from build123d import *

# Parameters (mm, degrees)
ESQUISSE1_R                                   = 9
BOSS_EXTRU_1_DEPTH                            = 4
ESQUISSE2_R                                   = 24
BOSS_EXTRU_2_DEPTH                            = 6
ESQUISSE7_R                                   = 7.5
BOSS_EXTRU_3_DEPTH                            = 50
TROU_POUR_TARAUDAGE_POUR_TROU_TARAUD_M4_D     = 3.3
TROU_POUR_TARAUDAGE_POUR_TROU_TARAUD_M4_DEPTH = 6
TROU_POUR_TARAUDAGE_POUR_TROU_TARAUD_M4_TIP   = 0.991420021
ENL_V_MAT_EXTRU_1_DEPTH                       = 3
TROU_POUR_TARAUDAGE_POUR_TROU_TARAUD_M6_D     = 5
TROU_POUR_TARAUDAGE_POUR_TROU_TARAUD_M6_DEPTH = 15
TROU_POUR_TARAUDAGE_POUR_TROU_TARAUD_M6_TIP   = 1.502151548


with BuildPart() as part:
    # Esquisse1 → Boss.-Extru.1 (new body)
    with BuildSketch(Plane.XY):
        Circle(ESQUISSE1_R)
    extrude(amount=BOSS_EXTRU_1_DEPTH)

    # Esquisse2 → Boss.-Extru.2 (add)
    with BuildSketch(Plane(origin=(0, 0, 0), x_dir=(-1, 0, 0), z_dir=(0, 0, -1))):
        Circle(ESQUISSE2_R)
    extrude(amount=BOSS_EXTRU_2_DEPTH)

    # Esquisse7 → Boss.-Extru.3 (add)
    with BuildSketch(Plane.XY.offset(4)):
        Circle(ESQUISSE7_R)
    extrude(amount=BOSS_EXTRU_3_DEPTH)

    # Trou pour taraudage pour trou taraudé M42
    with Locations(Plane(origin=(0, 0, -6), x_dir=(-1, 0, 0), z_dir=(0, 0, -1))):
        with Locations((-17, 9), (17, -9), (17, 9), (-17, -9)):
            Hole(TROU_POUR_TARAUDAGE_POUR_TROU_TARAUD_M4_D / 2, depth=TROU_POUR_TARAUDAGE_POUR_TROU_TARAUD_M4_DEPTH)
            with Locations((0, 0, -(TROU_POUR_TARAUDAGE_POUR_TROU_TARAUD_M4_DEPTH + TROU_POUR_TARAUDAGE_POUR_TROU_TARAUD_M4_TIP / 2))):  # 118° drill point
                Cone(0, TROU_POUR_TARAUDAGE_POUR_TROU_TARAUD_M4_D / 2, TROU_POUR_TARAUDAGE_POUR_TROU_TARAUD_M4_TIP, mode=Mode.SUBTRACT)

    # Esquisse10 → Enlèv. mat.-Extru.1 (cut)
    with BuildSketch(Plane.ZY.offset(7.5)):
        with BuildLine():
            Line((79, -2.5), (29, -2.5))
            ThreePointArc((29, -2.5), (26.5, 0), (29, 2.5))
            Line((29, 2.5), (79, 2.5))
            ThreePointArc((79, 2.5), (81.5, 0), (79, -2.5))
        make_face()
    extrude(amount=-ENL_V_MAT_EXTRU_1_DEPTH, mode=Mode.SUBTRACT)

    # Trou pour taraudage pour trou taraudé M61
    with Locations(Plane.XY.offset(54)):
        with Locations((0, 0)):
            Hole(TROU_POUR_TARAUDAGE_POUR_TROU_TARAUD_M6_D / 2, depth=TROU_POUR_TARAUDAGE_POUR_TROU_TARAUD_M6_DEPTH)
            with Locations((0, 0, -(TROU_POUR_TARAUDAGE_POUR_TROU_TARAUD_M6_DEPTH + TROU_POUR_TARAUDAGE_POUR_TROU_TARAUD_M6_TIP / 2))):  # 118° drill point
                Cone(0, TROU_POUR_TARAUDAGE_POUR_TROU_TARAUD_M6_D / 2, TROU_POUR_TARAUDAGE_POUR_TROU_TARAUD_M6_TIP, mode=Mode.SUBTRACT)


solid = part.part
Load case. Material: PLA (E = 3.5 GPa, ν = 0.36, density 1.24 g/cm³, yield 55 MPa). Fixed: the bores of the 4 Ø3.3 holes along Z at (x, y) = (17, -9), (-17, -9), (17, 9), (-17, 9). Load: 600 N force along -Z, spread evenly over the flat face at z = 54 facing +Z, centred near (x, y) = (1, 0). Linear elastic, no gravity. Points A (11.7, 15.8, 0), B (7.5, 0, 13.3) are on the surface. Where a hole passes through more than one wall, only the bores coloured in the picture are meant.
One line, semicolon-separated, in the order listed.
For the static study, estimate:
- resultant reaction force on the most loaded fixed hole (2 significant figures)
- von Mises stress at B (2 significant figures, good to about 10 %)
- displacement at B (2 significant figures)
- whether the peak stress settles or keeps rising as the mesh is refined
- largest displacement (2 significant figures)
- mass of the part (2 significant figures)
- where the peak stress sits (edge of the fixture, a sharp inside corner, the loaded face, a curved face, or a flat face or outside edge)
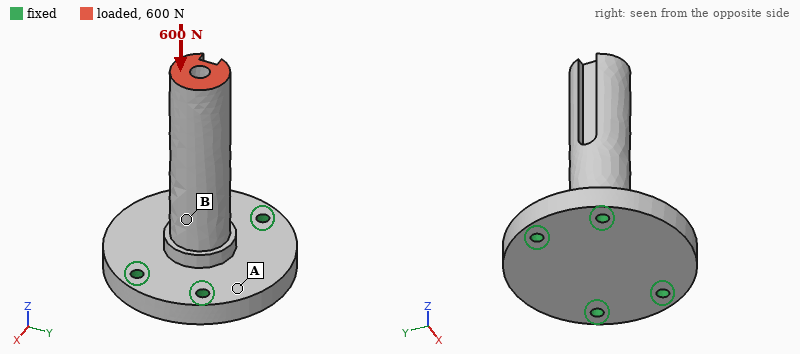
160 N; 4.5 MPa; 0.065 mm; keeps rising; 0.13 mm; 25 g; edge of the fixture
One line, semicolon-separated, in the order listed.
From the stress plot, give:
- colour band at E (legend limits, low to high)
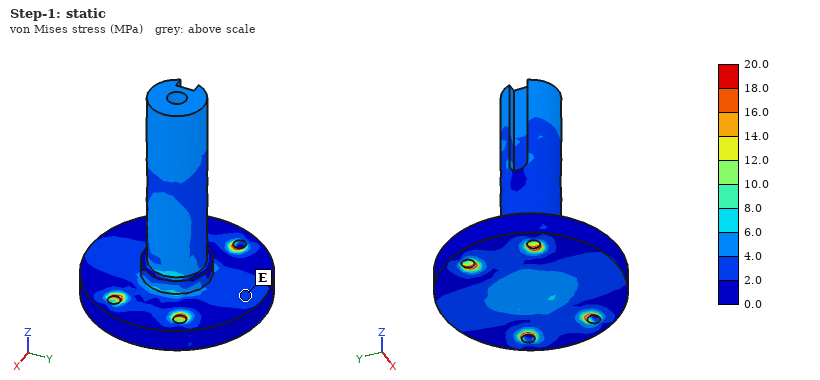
2.0 to 4.0 MPa
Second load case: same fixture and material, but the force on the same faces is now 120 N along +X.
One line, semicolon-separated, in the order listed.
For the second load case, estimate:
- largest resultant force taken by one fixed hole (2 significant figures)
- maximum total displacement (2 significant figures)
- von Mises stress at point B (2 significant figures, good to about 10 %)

130 N; 0.95 mm; 15 MPa
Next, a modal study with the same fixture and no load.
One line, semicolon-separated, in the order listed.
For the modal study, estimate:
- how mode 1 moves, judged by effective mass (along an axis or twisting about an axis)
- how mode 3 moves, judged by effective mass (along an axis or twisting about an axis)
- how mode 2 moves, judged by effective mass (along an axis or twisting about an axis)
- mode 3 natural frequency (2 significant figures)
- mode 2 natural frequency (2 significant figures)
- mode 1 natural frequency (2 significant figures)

along Y; along Z; along X; 4000 Hz; 1100 Hz; 1000 Hz
